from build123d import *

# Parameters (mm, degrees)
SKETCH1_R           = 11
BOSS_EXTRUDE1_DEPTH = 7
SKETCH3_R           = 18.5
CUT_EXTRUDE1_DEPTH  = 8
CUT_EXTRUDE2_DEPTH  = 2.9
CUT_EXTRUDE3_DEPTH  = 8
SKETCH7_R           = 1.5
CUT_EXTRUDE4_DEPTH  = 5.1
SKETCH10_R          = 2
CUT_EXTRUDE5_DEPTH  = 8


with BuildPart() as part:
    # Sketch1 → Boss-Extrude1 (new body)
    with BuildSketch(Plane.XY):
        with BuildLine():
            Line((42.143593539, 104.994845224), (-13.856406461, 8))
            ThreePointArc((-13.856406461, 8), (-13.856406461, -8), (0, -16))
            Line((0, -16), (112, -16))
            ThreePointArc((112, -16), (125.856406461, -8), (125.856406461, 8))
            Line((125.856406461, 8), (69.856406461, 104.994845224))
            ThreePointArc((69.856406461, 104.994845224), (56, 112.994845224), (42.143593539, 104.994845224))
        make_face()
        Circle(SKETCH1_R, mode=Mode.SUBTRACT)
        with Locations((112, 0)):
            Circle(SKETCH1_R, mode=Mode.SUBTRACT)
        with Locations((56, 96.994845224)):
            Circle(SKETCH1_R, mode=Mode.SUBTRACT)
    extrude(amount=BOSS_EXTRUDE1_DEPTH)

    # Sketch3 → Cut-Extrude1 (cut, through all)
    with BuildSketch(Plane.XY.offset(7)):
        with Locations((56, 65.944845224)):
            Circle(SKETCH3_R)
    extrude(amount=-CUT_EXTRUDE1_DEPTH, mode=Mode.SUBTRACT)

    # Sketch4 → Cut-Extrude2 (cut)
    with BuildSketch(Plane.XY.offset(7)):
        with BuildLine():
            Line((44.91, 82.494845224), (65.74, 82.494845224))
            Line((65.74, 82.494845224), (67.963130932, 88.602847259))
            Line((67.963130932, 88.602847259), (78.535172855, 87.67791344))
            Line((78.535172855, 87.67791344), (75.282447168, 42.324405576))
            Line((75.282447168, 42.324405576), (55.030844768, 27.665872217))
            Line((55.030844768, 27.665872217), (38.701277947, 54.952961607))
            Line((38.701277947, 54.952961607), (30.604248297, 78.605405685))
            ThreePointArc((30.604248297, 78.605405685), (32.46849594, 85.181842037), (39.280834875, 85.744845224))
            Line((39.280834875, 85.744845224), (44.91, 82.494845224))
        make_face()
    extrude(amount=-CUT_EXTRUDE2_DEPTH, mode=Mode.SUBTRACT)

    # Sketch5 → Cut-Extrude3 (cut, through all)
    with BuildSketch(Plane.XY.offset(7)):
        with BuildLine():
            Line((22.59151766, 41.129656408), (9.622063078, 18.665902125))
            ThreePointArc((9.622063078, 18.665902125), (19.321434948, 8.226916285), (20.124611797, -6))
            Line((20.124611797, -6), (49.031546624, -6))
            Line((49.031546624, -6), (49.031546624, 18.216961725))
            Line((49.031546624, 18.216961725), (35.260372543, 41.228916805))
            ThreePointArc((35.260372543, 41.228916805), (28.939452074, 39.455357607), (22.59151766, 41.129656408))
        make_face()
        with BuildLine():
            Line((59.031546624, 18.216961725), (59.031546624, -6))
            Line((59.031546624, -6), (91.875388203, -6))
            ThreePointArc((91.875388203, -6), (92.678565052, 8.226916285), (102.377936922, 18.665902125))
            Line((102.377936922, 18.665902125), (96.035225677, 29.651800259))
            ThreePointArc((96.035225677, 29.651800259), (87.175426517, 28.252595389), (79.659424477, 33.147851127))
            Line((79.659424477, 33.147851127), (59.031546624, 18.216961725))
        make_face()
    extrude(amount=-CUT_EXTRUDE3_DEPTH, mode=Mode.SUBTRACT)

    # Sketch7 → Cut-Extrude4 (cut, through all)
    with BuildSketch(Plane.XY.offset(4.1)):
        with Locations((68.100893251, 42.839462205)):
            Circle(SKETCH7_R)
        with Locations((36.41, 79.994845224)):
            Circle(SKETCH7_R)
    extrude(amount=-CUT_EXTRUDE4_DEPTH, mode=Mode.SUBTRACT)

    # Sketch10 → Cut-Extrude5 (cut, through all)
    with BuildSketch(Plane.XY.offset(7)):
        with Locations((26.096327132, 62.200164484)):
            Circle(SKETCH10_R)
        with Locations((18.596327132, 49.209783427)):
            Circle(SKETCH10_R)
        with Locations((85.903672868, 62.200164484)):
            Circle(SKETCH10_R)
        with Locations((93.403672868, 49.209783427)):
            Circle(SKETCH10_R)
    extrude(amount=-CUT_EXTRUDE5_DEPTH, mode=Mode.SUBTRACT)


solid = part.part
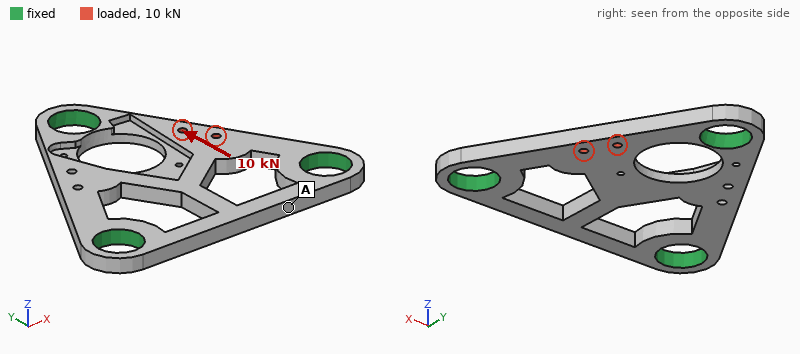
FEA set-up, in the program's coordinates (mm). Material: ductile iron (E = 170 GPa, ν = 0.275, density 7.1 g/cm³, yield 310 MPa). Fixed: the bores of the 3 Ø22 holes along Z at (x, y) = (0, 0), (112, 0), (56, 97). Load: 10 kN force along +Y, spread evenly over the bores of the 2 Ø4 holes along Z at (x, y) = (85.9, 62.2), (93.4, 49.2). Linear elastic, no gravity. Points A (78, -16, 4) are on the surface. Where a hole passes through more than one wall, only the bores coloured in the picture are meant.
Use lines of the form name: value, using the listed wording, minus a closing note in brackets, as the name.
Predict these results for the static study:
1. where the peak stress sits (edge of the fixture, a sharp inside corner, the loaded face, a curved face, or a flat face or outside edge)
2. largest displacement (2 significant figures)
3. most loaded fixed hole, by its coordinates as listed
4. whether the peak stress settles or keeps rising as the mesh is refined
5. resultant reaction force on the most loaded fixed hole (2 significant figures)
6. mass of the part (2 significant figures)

where the peak stress sits: a sharp inside corner
largest displacement: 33 µm
most loaded fixed hole, by its coordinates as listed: (112, 0)
whether the peak stress settles or keeps rising as the mesh is refined: keeps rising
resultant reaction force on the most loaded fixed hole: 5.0 kN
mass of the part: 320 g
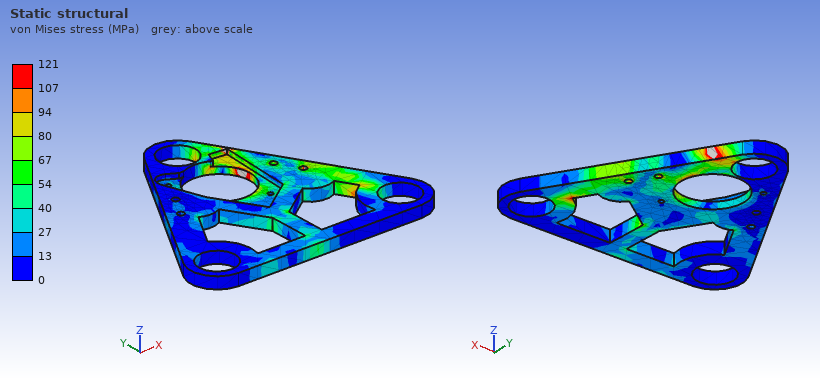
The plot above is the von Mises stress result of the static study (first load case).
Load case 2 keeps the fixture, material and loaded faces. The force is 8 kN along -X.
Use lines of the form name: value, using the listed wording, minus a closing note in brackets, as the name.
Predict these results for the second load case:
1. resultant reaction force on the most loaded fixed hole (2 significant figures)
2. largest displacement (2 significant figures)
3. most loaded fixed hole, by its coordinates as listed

resultant reaction force on the most loaded fixed hole: 3.5 kN
largest displacement: 47 µm
most loaded fixed hole, by its coordinates as listed: (112, 0)
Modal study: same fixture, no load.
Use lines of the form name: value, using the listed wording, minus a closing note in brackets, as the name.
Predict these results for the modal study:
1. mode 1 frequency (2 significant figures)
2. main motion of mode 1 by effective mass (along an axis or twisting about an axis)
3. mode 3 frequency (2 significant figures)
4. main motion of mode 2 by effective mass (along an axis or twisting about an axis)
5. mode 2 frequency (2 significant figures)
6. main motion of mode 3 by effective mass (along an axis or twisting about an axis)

mode 1 frequency: 2500 Hz
main motion of mode 1 by effective mass: along Z
mode 3 frequency: 3900 Hz
main motion of mode 2 by effective mass: twisting about Y
mode 2 frequency: 3700 Hz
main motion of mode 3 by effective mass: twisting about X
